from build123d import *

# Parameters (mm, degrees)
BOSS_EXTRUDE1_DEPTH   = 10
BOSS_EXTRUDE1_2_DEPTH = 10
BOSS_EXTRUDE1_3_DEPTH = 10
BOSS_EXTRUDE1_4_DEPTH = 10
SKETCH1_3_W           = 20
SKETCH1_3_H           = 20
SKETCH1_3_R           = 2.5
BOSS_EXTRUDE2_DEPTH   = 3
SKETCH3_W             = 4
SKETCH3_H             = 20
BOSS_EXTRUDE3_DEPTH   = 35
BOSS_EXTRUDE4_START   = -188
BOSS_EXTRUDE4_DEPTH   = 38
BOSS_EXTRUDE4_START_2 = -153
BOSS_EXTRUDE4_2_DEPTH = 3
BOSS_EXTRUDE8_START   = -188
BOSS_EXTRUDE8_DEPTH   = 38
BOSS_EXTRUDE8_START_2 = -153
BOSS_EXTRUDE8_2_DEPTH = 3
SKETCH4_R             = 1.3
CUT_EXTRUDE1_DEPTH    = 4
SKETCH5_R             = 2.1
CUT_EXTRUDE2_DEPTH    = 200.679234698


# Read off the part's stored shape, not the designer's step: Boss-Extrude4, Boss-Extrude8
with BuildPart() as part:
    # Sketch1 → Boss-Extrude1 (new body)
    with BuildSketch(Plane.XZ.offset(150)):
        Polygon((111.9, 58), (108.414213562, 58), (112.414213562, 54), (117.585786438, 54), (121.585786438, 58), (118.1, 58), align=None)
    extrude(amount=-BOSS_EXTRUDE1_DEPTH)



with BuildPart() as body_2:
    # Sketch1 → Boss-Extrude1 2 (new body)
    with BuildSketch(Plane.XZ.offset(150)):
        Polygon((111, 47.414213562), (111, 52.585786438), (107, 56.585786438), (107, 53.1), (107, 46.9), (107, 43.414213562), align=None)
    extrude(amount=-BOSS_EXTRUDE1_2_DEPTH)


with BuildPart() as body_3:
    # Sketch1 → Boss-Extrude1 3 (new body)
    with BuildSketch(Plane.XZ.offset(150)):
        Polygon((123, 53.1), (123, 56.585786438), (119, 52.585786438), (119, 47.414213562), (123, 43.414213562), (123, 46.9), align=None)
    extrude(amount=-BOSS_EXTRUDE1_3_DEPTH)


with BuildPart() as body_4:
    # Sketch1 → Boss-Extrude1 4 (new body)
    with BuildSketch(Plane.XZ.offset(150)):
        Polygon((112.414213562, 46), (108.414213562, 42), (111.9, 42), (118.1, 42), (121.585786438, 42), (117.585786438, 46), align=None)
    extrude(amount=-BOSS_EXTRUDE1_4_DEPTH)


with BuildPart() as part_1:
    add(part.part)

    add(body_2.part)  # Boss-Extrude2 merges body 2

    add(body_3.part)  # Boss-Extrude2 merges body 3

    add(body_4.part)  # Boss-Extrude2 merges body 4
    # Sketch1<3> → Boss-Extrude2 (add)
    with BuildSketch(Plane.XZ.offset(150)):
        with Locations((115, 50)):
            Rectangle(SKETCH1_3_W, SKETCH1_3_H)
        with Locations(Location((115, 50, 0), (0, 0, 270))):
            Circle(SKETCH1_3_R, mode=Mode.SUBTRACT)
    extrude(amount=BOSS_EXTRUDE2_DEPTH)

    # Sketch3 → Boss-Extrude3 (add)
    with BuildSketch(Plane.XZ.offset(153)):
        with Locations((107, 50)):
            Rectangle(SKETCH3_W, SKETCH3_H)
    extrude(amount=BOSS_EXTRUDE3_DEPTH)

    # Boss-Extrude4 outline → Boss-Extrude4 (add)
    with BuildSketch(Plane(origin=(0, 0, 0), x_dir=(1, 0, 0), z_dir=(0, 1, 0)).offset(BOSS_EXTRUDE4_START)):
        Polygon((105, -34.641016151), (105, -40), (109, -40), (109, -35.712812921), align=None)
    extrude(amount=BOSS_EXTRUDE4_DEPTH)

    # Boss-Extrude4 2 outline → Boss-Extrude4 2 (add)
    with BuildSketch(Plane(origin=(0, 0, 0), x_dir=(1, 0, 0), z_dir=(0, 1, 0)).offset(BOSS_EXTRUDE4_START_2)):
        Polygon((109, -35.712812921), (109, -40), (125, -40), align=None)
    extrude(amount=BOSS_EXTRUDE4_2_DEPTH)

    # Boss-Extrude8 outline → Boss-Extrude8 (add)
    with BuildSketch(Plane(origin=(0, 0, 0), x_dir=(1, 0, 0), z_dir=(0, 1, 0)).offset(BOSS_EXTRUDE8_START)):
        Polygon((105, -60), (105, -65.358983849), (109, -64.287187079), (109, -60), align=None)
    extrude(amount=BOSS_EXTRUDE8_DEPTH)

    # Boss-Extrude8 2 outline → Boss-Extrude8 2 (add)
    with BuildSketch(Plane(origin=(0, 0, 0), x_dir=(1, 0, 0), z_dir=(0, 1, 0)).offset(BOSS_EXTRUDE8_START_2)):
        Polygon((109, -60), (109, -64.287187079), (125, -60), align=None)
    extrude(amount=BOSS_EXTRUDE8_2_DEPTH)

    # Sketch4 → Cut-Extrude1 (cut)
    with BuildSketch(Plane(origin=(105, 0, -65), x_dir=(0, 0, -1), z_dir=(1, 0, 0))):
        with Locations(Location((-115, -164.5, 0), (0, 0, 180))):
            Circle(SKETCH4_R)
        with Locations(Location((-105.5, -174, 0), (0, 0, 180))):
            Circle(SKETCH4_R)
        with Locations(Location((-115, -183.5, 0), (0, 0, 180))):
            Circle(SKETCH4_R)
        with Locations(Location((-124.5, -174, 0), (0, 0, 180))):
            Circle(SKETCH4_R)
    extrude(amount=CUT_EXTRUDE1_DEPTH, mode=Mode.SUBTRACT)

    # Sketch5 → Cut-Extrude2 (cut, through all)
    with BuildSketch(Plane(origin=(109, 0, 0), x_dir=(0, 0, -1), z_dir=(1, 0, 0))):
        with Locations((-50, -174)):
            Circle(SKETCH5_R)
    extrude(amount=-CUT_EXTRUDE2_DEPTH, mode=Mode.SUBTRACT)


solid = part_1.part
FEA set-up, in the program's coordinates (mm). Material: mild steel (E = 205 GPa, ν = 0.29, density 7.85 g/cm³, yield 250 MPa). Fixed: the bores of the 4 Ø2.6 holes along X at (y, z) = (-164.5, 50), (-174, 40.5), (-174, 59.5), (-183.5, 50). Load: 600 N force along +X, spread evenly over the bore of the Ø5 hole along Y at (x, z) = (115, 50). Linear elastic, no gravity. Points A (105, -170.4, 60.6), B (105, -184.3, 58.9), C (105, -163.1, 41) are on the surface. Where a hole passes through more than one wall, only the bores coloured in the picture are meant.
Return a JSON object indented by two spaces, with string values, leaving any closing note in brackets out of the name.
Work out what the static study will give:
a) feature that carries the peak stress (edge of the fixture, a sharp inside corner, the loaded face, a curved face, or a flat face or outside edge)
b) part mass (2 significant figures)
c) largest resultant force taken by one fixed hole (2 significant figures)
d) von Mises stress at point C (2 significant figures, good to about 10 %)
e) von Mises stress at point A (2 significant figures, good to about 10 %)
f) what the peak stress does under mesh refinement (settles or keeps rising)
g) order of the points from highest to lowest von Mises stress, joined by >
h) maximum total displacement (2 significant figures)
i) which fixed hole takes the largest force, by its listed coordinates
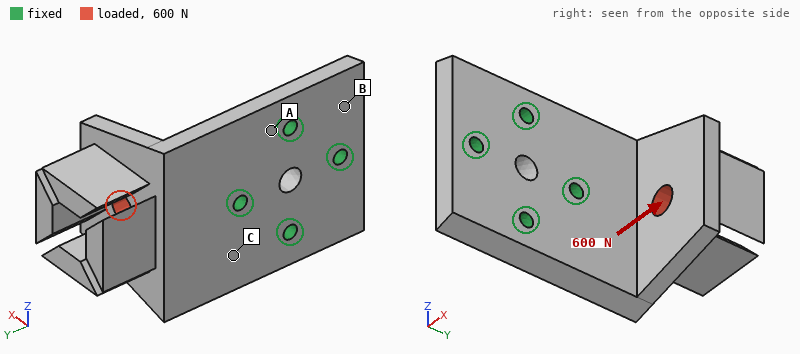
{
  "feature that carries the peak stress": "edge of the fixture",
  "part mass": "54 g",
  "largest resultant force taken by one fixed hole": "890 N",
  "von Mises stress at point C": "53 MPa",
  "von Mises stress at point A": "28 MPa",
  "what the peak stress does under mesh refinement": "keeps rising",
  "order of the points from highest to lowest von Mises stress, joined by >": "C > A > B",
  "maximum total displacement": "53 µm",
  "which fixed hole takes the largest force, by its listed coordinates": "(-164.5, 50)"
}
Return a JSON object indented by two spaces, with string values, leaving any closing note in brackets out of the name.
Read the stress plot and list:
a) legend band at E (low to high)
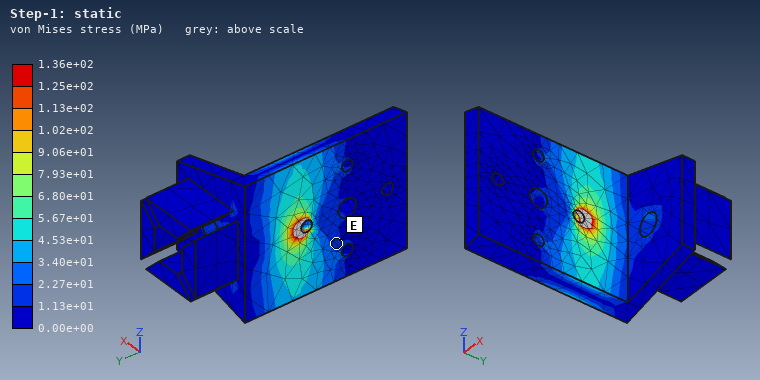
{
  "legend band at E": "1.13e+01 to 2.27e+01 MPa"
}
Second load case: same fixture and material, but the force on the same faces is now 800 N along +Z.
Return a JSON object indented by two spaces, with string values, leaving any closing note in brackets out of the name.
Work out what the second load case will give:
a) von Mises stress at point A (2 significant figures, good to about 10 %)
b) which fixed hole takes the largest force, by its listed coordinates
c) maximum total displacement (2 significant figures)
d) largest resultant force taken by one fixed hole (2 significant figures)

{
  "von Mises stress at point A": "63 MPa",
  "which fixed hole takes the largest force, by its listed coordinates": "(-164.5, 50)",
  "maximum total displacement": "36 µm",
  "largest resultant force taken by one fixed hole": "850 N"
}
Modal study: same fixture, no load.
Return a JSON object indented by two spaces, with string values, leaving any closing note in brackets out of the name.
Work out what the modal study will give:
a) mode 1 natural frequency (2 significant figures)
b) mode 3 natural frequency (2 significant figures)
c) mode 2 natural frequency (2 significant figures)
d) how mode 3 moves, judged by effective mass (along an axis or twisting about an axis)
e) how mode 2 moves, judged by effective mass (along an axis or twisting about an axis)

{
  "mode 1 natural frequency": "3000 Hz",
  "mode 3 natural frequency": "9500 Hz",
  "mode 2 natural frequency": "5500 Hz",
  "how mode 3 moves, judged by effective mass": "along X",
  "how mode 2 moves, judged by effective mass": "along Z"
}
